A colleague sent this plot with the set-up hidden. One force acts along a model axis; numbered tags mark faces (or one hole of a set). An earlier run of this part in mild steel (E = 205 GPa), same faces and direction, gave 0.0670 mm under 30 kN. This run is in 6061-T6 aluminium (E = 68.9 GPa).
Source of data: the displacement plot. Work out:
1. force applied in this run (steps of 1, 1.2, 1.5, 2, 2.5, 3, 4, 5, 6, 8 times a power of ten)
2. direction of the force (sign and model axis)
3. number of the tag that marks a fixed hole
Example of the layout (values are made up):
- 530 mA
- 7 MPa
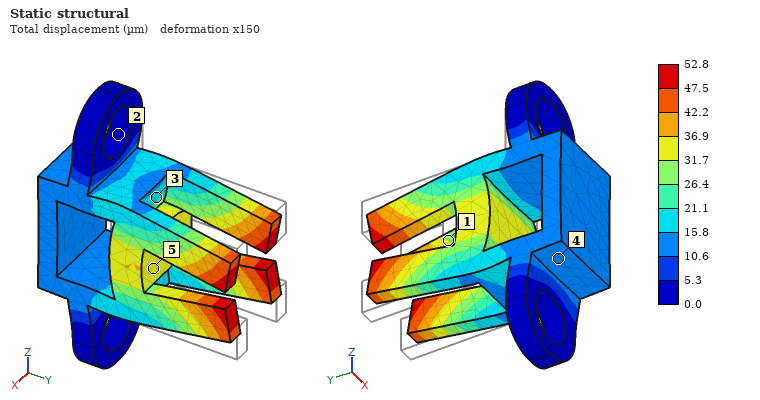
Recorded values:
- 8 kN
- -Y
- 2
